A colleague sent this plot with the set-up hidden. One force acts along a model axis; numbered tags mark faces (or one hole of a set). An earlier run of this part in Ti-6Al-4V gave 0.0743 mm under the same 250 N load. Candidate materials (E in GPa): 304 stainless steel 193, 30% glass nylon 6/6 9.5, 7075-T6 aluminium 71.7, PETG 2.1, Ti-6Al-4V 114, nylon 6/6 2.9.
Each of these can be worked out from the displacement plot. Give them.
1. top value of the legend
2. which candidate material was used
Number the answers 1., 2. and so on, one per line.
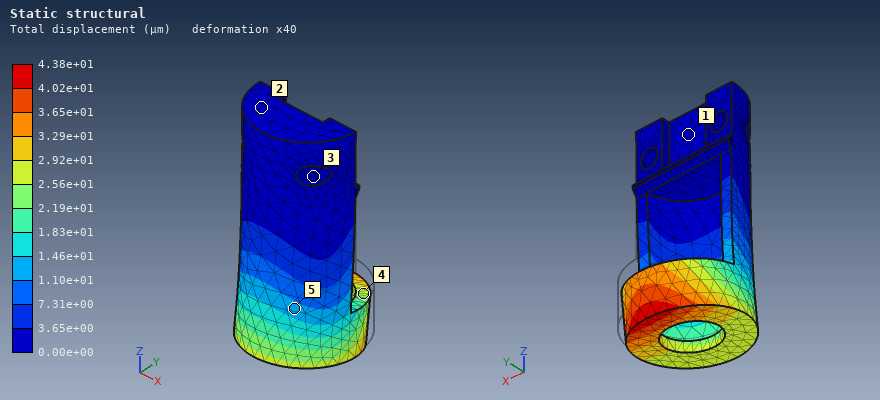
1. 4.38e+01 µm
2. 304 stainless steel
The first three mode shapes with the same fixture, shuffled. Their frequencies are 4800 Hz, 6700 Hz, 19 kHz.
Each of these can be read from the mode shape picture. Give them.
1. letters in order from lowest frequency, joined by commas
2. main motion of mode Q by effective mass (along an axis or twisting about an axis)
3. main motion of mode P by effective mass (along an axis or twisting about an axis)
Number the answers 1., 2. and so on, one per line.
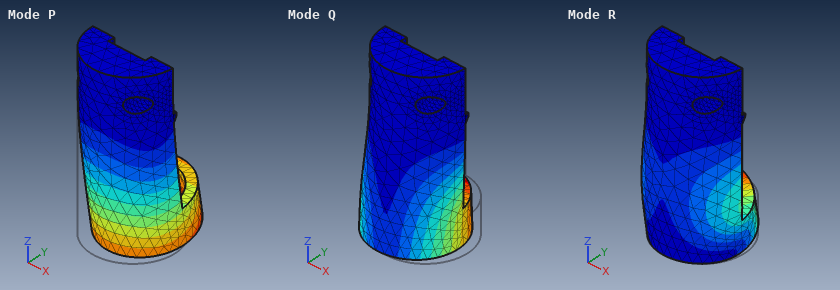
1. Q, P, R
2. along X
3. along Y
